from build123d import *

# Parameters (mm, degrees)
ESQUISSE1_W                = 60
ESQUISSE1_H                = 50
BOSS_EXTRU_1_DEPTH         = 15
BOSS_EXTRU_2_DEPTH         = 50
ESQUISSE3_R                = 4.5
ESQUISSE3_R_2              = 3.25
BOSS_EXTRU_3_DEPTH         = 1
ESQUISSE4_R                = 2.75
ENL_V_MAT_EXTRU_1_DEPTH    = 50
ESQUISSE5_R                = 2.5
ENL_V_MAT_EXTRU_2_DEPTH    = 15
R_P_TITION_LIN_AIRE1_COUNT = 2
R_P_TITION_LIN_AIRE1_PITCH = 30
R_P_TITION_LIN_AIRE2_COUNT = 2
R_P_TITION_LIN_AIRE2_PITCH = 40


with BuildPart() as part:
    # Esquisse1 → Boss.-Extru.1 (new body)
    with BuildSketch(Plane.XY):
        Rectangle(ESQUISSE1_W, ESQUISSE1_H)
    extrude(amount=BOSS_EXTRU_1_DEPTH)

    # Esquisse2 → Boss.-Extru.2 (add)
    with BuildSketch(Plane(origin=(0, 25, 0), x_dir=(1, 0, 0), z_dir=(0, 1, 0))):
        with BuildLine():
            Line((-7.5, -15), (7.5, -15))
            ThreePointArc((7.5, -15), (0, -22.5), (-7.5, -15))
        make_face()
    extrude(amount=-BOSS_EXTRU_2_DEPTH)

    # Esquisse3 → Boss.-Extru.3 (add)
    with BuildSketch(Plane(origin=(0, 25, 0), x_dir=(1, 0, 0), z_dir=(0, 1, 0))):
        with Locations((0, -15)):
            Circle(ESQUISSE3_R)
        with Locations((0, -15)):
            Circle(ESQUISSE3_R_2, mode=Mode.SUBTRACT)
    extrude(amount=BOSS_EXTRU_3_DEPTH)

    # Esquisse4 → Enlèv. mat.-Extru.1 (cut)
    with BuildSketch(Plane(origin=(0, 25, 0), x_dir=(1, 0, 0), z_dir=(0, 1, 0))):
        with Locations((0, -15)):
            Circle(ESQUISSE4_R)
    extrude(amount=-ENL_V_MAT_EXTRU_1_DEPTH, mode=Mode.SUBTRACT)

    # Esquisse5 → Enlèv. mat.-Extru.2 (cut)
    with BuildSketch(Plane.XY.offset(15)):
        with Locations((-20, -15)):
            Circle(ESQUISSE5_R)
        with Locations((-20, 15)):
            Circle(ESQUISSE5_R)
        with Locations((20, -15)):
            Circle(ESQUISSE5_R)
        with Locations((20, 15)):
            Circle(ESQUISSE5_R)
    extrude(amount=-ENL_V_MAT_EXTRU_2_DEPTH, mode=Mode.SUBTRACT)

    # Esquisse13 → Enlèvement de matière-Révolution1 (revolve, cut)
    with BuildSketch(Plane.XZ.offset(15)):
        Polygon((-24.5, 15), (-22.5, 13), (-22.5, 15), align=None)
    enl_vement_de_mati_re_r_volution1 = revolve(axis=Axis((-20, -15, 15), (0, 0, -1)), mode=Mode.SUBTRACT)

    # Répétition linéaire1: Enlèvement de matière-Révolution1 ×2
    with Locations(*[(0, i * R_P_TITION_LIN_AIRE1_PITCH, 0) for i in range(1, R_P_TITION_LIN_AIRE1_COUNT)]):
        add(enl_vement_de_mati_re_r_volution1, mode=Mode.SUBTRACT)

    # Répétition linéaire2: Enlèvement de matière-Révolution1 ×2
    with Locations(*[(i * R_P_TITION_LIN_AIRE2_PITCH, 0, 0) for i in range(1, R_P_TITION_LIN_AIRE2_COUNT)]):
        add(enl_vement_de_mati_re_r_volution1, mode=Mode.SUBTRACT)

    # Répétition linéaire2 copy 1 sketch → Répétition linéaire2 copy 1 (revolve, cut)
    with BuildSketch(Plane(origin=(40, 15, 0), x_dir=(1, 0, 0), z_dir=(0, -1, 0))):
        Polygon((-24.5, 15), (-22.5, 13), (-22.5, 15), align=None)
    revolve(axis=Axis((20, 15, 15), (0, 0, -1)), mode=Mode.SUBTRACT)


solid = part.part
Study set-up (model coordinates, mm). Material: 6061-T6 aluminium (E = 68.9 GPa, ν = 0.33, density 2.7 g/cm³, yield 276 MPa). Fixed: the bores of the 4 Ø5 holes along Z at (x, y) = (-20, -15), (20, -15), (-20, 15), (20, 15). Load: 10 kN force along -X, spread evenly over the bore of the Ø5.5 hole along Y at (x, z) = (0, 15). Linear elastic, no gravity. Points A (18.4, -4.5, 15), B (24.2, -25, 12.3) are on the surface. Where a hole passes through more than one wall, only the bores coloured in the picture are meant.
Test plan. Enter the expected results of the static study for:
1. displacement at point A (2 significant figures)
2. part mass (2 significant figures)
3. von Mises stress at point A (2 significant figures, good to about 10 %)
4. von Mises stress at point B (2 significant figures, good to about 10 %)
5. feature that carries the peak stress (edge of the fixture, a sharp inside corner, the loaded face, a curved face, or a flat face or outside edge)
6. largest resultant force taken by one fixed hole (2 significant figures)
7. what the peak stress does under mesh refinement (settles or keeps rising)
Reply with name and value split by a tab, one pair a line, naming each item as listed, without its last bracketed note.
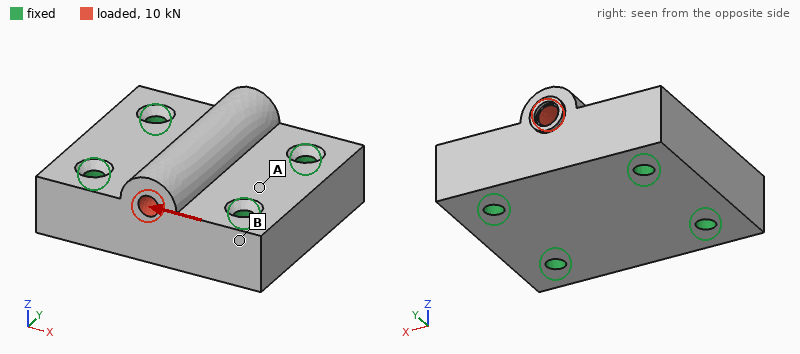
displacement at point A	1.7 µm
part mass	130 g
von Mises stress at point A	4.9 MPa
von Mises stress at point B	2.7 MPa
feature that carries the peak stress	edge of the fixture
largest resultant force taken by one fixed hole	2.7 kN
what the peak stress does under mesh refinement	keeps rising
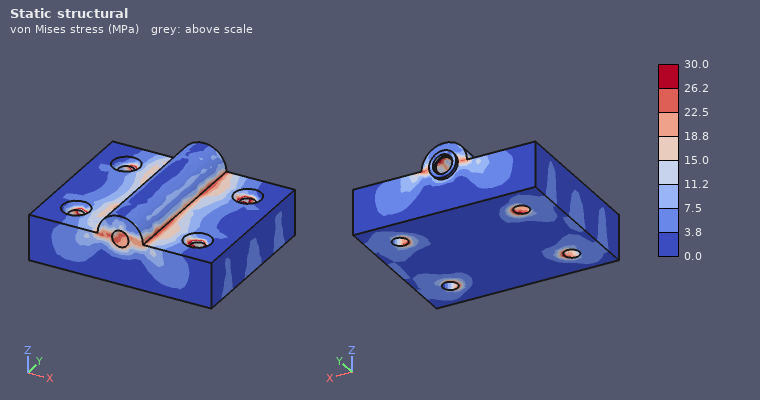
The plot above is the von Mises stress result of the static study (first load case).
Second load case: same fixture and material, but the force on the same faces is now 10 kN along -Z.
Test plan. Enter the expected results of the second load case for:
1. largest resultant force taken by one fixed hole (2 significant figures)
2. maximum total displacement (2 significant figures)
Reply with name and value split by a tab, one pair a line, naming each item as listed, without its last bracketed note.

largest resultant force taken by one fixed hole	2.6 kN
maximum total displacement	10 µm
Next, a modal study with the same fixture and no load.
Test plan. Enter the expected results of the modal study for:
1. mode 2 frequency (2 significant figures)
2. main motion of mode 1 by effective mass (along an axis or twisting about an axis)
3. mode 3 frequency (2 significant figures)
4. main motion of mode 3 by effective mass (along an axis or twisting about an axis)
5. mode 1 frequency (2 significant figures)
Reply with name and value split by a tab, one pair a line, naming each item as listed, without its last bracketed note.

mode 2 frequency	25 kHz
main motion of mode 1 by effective mass	along Z
mode 3 frequency	31 kHz
main motion of mode 3 by effective mass	along Y
mode 1 frequency	23 kHz
